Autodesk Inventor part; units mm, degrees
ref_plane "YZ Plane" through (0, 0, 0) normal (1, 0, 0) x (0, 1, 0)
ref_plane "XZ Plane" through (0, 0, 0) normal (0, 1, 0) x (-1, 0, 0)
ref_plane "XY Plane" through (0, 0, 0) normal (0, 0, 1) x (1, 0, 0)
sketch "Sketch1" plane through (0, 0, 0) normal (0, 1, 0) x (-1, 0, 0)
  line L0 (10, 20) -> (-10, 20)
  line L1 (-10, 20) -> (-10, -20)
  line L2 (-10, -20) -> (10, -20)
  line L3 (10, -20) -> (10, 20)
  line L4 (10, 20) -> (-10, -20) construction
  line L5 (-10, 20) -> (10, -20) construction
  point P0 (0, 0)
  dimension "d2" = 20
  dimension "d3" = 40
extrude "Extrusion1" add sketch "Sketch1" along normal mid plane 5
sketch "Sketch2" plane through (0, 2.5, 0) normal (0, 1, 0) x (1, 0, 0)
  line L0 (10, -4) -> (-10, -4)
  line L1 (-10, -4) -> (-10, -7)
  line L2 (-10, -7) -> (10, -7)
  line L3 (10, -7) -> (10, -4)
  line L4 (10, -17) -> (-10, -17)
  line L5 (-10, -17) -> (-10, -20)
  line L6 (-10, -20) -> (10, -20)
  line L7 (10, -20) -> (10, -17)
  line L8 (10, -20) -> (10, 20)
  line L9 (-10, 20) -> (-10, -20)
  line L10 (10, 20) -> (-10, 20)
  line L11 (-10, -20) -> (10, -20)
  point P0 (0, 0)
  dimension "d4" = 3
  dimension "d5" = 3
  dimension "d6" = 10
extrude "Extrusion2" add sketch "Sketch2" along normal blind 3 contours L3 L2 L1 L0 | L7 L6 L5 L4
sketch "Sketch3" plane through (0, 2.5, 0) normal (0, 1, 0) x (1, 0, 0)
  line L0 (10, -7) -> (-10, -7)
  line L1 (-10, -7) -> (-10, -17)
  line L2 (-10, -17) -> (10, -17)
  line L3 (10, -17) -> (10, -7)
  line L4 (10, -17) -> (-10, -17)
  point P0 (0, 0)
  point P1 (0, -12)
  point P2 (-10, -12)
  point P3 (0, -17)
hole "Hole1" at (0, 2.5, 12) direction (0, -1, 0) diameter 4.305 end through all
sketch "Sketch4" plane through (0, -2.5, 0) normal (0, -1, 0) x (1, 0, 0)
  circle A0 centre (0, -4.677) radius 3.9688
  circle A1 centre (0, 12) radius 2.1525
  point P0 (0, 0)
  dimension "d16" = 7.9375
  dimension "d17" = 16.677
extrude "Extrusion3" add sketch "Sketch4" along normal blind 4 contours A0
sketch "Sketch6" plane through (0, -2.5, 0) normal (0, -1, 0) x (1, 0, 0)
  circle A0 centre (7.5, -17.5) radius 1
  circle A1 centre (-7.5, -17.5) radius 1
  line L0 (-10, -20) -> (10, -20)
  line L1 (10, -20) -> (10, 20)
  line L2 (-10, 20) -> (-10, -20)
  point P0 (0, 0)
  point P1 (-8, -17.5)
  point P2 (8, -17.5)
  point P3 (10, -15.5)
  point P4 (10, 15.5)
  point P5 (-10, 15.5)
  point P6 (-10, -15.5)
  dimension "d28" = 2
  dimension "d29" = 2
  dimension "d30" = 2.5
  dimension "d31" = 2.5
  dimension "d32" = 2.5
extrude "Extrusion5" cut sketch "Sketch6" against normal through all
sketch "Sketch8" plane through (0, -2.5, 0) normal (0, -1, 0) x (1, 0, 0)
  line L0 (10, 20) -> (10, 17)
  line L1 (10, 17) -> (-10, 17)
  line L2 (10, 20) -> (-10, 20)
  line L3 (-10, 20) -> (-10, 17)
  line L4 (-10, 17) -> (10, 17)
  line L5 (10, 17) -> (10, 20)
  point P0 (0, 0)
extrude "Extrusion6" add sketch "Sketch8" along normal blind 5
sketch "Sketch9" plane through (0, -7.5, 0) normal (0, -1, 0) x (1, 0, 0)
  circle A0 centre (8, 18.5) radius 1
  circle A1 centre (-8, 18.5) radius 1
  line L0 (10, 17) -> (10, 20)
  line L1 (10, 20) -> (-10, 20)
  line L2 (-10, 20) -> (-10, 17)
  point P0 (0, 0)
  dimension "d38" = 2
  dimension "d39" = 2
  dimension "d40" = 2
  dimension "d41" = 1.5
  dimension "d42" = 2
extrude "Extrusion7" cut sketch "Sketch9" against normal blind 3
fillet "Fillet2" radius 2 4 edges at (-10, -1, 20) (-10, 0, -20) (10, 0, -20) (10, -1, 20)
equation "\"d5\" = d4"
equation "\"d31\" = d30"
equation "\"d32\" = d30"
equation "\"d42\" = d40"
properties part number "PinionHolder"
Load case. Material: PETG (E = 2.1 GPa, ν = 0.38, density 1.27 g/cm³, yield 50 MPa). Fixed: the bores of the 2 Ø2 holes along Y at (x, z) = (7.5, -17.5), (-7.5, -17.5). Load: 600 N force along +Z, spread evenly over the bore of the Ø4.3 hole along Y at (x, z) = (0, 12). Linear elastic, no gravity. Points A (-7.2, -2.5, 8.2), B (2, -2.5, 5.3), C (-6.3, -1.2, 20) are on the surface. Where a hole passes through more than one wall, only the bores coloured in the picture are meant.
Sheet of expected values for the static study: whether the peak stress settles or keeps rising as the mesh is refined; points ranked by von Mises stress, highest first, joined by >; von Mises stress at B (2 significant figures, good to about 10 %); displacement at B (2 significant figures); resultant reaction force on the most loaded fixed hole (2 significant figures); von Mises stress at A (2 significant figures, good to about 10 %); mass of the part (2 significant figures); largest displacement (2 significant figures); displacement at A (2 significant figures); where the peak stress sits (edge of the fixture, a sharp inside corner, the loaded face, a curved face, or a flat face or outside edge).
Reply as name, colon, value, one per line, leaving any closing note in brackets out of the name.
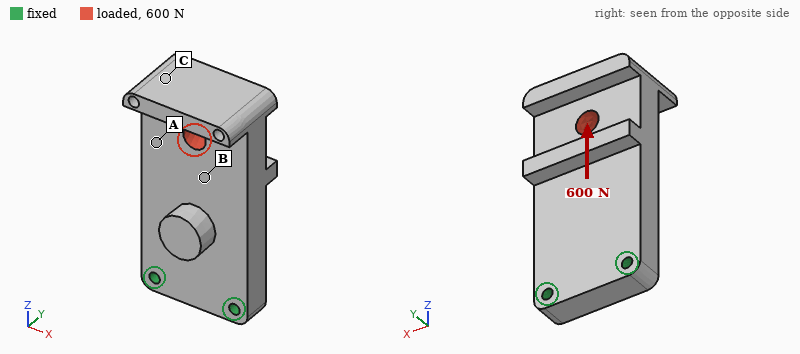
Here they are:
whether the peak stress settles or keeps rising as the mesh is refined: keeps rising
points ranked by von Mises stress, highest first, joined by >: B > A > C
von Mises stress at B: 8.4 MPa
displacement at B: 0.077 mm
resultant reaction force on the most loaded fixed hole: 310 N
von Mises stress at A: 4.9 MPa
mass of the part: 6.0 g
largest displacement: 0.12 mm
displacement at A: 0.080 mm
where the peak stress sits: edge of the fixture
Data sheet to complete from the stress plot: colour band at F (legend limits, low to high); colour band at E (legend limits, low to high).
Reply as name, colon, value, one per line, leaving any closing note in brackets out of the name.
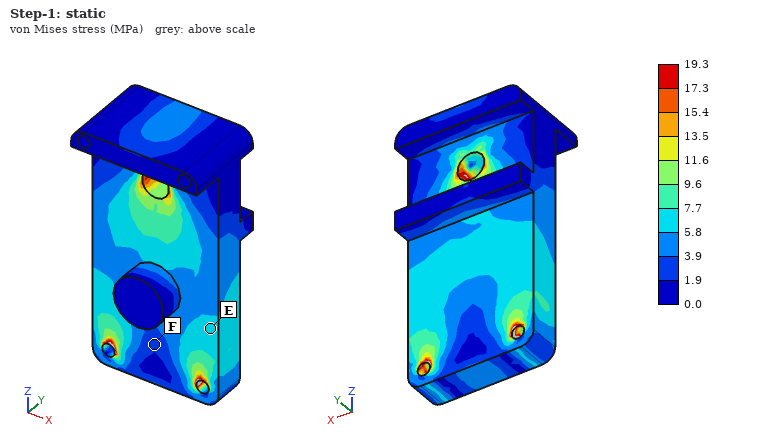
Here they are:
colour band at F: 1.9 to 3.9 MPa
colour band at E: 5.8 to 7.7 MPa
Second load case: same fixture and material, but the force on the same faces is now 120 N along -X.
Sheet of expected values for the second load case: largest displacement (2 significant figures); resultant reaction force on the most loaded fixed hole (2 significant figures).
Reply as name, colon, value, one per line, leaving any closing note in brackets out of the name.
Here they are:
largest displacement: 0.27 mm
resultant reaction force on the most loaded fixed hole: 230 N
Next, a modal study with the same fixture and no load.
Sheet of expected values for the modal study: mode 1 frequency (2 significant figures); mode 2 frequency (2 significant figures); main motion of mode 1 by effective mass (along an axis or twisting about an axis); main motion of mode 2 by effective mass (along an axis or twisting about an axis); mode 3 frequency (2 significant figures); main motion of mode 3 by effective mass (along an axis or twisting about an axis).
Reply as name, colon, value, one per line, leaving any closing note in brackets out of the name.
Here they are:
mode 1 frequency: 580 Hz
mode 2 frequency: 2100 Hz
main motion of mode 1 by effective mass: along Y
main motion of mode 2 by effective mass: along X
mode 3 frequency: 2200 Hz
main motion of mode 3 by effective mass: twisting about Z
